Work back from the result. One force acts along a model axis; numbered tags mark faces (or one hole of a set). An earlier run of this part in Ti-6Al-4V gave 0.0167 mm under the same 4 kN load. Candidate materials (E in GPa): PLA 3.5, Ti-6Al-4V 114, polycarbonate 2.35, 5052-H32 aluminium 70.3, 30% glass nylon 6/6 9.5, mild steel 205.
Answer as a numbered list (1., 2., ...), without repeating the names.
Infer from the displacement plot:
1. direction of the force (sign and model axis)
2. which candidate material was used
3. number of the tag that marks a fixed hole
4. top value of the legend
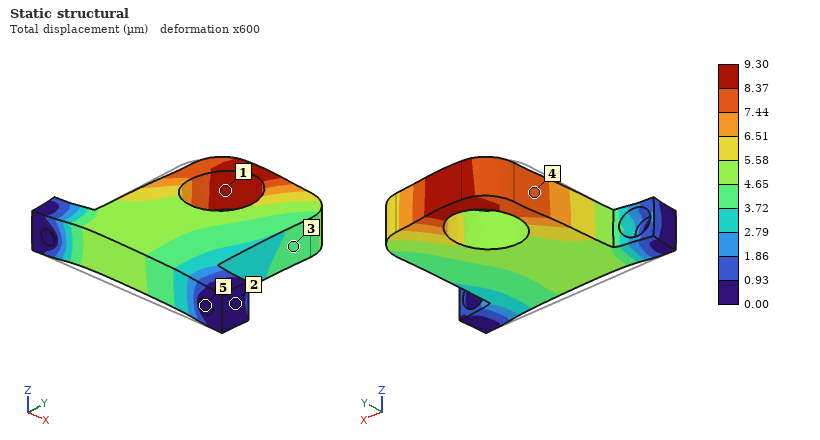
1. +Y
2. mild steel
3. 5
4. 9.30 µm
